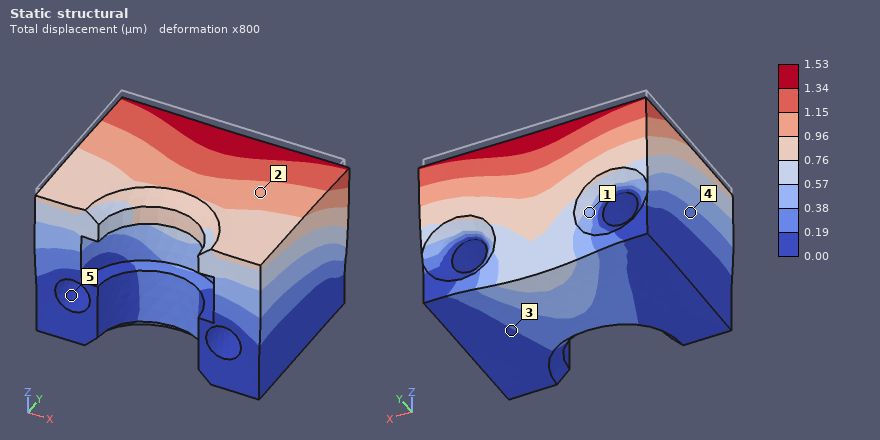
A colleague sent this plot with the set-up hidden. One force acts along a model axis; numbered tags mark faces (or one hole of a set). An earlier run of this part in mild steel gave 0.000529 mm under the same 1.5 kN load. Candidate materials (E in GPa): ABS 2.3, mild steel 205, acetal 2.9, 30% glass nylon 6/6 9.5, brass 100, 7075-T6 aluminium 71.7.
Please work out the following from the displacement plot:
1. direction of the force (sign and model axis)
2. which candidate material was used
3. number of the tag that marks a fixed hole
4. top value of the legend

-Z
7075-T6 aluminium
5
1.53 µm
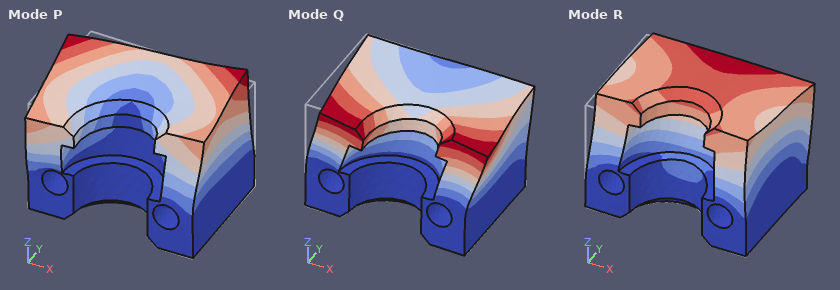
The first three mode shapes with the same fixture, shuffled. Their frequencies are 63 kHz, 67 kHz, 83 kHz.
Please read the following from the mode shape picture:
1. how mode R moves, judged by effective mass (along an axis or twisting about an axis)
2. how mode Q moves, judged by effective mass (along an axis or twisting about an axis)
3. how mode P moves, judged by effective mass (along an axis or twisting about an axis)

along Y
along X
along X
